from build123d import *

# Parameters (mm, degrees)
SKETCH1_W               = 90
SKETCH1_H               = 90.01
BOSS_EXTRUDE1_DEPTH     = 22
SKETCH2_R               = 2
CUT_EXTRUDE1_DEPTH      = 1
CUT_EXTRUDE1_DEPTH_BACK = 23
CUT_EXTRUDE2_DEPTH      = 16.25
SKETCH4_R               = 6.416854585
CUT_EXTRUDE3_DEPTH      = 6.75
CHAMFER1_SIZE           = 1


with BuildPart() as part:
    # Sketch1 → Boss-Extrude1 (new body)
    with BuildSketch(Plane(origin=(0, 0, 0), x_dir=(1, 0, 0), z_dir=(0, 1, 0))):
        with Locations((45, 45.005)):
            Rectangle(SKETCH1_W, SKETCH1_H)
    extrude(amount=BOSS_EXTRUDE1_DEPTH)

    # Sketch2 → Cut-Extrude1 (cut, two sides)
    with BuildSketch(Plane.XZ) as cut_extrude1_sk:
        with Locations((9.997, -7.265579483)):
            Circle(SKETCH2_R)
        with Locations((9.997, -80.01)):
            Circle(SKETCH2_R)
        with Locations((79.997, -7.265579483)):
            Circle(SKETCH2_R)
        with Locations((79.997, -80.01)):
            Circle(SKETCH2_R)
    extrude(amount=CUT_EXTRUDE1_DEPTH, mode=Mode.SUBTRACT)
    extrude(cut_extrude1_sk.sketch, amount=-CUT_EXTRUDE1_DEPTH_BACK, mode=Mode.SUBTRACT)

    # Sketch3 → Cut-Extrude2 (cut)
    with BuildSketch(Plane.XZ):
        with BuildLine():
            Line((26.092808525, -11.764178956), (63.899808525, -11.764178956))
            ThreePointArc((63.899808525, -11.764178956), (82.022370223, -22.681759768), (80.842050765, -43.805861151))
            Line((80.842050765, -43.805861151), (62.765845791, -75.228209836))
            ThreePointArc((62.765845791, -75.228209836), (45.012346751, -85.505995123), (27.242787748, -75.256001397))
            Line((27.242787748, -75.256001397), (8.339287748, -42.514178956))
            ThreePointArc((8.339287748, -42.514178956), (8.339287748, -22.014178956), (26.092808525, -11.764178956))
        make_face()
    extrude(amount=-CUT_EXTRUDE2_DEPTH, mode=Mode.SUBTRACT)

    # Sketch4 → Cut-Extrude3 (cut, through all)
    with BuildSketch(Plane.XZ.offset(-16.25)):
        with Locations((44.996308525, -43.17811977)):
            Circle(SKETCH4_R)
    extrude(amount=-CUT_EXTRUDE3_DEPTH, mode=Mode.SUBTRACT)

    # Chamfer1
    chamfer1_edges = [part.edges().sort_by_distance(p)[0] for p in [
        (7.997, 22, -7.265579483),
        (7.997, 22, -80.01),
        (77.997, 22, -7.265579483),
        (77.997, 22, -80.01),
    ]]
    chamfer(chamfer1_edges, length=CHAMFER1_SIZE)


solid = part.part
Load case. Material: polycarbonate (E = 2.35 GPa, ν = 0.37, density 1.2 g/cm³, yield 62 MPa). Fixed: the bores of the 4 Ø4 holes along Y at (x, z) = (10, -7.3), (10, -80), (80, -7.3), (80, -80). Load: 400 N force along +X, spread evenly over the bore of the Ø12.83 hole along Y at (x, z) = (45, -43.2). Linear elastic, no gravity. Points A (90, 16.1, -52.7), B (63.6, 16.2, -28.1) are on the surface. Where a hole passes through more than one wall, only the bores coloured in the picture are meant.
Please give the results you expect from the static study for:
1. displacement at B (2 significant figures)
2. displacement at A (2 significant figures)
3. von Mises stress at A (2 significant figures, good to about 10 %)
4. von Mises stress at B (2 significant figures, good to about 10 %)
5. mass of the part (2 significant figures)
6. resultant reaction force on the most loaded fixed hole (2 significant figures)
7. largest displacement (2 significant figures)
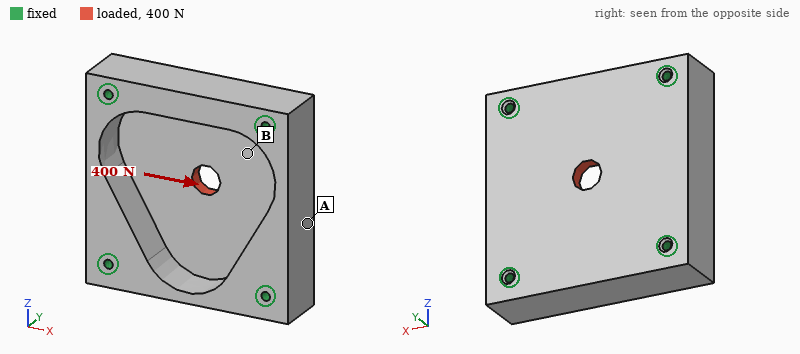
12 µm
9.6 µm
0.35 MPa
0.90 MPa
130 g
110 N
23 µm
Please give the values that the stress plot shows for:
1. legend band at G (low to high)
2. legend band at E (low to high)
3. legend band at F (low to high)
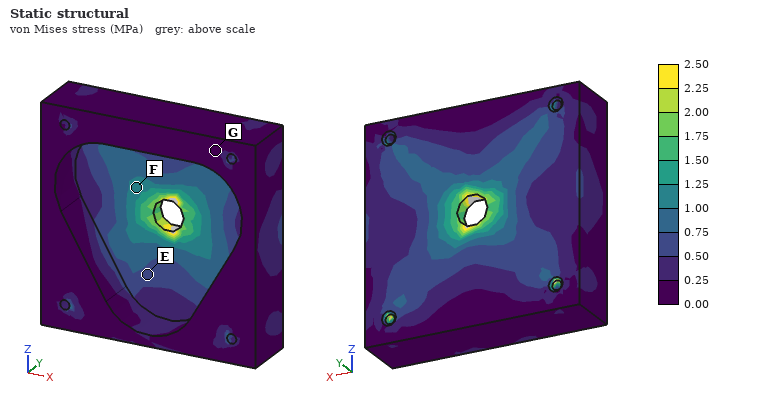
0.00 to 0.25 MPa
0.50 to 0.75 MPa
1.00 to 1.25 MPa
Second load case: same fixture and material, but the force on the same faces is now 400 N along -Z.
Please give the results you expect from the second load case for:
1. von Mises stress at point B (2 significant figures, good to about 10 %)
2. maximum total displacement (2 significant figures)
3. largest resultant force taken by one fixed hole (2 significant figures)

0.84 MPa
23 µm
120 N
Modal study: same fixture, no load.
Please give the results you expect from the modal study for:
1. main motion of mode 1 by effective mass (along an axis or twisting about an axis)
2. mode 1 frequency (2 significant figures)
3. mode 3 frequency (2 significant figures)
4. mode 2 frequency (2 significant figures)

along Y
2300 Hz
3600 Hz
3500 Hz
